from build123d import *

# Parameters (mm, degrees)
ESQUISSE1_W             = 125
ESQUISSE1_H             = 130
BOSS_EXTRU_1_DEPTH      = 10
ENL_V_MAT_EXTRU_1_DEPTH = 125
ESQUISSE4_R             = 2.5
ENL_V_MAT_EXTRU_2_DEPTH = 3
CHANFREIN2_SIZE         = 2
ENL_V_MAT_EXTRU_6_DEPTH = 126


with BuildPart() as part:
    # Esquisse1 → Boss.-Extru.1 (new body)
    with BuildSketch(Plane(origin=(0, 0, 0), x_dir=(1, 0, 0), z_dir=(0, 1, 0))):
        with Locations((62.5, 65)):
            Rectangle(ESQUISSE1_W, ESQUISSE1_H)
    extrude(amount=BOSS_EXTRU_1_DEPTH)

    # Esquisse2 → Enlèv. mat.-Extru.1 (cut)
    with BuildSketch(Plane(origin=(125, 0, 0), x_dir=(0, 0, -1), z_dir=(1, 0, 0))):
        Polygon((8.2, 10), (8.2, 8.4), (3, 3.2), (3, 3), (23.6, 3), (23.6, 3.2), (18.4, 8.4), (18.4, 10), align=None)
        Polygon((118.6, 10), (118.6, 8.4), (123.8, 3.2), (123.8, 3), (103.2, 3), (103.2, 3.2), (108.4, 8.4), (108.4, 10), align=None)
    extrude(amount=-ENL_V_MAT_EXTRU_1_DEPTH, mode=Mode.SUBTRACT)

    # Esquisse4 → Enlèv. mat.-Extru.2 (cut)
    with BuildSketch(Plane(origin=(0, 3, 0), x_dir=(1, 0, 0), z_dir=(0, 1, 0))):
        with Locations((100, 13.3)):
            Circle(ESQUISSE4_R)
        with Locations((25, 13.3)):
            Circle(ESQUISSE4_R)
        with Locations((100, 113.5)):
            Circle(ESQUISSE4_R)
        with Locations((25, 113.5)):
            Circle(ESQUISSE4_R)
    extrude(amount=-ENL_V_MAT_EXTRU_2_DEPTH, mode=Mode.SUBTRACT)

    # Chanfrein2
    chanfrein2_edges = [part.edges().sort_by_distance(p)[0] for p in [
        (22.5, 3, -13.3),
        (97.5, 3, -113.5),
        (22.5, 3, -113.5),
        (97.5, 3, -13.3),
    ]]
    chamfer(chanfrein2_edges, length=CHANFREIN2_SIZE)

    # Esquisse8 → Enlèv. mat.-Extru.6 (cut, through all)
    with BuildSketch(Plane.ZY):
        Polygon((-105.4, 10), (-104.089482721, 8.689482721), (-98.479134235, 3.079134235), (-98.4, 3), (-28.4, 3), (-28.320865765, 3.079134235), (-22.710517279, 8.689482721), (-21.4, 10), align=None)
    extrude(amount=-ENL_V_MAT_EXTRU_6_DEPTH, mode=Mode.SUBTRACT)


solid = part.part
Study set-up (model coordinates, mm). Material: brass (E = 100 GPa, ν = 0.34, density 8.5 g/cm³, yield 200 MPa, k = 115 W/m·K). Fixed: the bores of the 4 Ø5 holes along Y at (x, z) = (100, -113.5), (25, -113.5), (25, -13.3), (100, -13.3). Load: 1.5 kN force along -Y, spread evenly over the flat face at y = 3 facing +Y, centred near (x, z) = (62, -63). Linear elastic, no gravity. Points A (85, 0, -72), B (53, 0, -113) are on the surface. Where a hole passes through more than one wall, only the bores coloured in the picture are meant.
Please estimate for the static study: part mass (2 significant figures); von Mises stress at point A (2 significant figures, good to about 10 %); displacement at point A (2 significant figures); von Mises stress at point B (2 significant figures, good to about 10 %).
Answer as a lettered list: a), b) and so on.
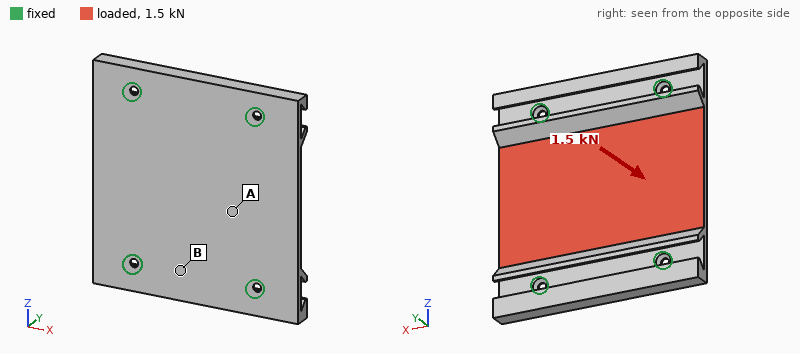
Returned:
a) 590 g
b) 46 MPa
c) 0.30 mm
d) 21 MPa
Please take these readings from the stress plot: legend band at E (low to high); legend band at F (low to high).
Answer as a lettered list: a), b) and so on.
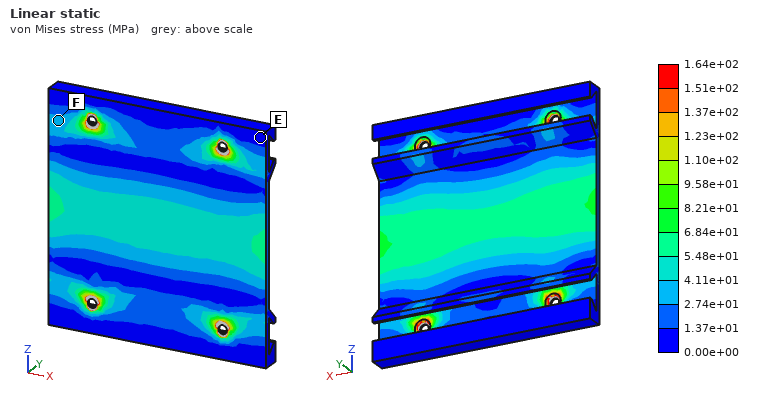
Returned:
a) 0.00e+00 to 1.37e+01 MPa
b) 2.74e+01 to 4.11e+01 MPa
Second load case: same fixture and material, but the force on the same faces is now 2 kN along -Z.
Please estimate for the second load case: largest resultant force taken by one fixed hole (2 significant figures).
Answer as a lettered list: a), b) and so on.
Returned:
a) 510 N
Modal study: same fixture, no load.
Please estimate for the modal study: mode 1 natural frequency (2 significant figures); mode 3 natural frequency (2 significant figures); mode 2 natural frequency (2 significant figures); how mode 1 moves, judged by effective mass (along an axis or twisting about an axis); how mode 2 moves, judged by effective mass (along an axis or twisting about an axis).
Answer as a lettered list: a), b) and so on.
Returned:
a) 770 Hz
b) 1700 Hz
c) 1000 Hz
d) along Y
e) twisting about Z
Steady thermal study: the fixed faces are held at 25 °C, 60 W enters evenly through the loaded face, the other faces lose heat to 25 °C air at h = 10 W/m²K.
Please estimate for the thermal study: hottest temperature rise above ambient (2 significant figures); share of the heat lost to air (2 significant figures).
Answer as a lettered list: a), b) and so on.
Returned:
a) 34 K
b) 11 %
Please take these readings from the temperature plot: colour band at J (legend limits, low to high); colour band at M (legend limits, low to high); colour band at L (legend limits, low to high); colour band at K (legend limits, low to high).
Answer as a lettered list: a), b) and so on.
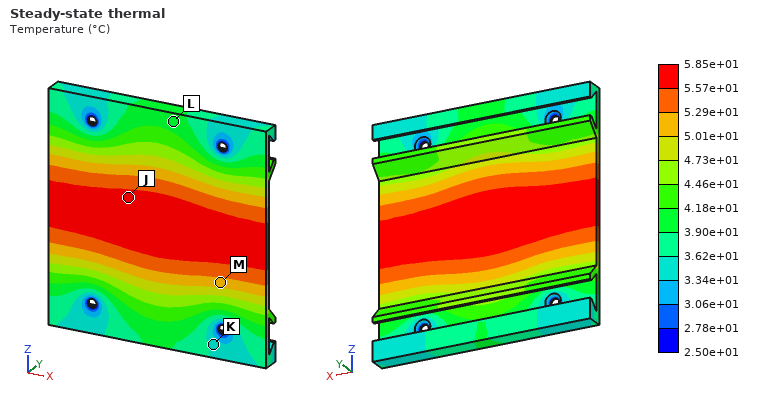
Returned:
a) 5.57e+01 to 5.85e+01 °C
b) 5.01e+01 to 5.29e+01 °C
c) 3.90e+01 to 4.18e+01 °C
d) 3.34e+01 to 3.62e+01 °C
